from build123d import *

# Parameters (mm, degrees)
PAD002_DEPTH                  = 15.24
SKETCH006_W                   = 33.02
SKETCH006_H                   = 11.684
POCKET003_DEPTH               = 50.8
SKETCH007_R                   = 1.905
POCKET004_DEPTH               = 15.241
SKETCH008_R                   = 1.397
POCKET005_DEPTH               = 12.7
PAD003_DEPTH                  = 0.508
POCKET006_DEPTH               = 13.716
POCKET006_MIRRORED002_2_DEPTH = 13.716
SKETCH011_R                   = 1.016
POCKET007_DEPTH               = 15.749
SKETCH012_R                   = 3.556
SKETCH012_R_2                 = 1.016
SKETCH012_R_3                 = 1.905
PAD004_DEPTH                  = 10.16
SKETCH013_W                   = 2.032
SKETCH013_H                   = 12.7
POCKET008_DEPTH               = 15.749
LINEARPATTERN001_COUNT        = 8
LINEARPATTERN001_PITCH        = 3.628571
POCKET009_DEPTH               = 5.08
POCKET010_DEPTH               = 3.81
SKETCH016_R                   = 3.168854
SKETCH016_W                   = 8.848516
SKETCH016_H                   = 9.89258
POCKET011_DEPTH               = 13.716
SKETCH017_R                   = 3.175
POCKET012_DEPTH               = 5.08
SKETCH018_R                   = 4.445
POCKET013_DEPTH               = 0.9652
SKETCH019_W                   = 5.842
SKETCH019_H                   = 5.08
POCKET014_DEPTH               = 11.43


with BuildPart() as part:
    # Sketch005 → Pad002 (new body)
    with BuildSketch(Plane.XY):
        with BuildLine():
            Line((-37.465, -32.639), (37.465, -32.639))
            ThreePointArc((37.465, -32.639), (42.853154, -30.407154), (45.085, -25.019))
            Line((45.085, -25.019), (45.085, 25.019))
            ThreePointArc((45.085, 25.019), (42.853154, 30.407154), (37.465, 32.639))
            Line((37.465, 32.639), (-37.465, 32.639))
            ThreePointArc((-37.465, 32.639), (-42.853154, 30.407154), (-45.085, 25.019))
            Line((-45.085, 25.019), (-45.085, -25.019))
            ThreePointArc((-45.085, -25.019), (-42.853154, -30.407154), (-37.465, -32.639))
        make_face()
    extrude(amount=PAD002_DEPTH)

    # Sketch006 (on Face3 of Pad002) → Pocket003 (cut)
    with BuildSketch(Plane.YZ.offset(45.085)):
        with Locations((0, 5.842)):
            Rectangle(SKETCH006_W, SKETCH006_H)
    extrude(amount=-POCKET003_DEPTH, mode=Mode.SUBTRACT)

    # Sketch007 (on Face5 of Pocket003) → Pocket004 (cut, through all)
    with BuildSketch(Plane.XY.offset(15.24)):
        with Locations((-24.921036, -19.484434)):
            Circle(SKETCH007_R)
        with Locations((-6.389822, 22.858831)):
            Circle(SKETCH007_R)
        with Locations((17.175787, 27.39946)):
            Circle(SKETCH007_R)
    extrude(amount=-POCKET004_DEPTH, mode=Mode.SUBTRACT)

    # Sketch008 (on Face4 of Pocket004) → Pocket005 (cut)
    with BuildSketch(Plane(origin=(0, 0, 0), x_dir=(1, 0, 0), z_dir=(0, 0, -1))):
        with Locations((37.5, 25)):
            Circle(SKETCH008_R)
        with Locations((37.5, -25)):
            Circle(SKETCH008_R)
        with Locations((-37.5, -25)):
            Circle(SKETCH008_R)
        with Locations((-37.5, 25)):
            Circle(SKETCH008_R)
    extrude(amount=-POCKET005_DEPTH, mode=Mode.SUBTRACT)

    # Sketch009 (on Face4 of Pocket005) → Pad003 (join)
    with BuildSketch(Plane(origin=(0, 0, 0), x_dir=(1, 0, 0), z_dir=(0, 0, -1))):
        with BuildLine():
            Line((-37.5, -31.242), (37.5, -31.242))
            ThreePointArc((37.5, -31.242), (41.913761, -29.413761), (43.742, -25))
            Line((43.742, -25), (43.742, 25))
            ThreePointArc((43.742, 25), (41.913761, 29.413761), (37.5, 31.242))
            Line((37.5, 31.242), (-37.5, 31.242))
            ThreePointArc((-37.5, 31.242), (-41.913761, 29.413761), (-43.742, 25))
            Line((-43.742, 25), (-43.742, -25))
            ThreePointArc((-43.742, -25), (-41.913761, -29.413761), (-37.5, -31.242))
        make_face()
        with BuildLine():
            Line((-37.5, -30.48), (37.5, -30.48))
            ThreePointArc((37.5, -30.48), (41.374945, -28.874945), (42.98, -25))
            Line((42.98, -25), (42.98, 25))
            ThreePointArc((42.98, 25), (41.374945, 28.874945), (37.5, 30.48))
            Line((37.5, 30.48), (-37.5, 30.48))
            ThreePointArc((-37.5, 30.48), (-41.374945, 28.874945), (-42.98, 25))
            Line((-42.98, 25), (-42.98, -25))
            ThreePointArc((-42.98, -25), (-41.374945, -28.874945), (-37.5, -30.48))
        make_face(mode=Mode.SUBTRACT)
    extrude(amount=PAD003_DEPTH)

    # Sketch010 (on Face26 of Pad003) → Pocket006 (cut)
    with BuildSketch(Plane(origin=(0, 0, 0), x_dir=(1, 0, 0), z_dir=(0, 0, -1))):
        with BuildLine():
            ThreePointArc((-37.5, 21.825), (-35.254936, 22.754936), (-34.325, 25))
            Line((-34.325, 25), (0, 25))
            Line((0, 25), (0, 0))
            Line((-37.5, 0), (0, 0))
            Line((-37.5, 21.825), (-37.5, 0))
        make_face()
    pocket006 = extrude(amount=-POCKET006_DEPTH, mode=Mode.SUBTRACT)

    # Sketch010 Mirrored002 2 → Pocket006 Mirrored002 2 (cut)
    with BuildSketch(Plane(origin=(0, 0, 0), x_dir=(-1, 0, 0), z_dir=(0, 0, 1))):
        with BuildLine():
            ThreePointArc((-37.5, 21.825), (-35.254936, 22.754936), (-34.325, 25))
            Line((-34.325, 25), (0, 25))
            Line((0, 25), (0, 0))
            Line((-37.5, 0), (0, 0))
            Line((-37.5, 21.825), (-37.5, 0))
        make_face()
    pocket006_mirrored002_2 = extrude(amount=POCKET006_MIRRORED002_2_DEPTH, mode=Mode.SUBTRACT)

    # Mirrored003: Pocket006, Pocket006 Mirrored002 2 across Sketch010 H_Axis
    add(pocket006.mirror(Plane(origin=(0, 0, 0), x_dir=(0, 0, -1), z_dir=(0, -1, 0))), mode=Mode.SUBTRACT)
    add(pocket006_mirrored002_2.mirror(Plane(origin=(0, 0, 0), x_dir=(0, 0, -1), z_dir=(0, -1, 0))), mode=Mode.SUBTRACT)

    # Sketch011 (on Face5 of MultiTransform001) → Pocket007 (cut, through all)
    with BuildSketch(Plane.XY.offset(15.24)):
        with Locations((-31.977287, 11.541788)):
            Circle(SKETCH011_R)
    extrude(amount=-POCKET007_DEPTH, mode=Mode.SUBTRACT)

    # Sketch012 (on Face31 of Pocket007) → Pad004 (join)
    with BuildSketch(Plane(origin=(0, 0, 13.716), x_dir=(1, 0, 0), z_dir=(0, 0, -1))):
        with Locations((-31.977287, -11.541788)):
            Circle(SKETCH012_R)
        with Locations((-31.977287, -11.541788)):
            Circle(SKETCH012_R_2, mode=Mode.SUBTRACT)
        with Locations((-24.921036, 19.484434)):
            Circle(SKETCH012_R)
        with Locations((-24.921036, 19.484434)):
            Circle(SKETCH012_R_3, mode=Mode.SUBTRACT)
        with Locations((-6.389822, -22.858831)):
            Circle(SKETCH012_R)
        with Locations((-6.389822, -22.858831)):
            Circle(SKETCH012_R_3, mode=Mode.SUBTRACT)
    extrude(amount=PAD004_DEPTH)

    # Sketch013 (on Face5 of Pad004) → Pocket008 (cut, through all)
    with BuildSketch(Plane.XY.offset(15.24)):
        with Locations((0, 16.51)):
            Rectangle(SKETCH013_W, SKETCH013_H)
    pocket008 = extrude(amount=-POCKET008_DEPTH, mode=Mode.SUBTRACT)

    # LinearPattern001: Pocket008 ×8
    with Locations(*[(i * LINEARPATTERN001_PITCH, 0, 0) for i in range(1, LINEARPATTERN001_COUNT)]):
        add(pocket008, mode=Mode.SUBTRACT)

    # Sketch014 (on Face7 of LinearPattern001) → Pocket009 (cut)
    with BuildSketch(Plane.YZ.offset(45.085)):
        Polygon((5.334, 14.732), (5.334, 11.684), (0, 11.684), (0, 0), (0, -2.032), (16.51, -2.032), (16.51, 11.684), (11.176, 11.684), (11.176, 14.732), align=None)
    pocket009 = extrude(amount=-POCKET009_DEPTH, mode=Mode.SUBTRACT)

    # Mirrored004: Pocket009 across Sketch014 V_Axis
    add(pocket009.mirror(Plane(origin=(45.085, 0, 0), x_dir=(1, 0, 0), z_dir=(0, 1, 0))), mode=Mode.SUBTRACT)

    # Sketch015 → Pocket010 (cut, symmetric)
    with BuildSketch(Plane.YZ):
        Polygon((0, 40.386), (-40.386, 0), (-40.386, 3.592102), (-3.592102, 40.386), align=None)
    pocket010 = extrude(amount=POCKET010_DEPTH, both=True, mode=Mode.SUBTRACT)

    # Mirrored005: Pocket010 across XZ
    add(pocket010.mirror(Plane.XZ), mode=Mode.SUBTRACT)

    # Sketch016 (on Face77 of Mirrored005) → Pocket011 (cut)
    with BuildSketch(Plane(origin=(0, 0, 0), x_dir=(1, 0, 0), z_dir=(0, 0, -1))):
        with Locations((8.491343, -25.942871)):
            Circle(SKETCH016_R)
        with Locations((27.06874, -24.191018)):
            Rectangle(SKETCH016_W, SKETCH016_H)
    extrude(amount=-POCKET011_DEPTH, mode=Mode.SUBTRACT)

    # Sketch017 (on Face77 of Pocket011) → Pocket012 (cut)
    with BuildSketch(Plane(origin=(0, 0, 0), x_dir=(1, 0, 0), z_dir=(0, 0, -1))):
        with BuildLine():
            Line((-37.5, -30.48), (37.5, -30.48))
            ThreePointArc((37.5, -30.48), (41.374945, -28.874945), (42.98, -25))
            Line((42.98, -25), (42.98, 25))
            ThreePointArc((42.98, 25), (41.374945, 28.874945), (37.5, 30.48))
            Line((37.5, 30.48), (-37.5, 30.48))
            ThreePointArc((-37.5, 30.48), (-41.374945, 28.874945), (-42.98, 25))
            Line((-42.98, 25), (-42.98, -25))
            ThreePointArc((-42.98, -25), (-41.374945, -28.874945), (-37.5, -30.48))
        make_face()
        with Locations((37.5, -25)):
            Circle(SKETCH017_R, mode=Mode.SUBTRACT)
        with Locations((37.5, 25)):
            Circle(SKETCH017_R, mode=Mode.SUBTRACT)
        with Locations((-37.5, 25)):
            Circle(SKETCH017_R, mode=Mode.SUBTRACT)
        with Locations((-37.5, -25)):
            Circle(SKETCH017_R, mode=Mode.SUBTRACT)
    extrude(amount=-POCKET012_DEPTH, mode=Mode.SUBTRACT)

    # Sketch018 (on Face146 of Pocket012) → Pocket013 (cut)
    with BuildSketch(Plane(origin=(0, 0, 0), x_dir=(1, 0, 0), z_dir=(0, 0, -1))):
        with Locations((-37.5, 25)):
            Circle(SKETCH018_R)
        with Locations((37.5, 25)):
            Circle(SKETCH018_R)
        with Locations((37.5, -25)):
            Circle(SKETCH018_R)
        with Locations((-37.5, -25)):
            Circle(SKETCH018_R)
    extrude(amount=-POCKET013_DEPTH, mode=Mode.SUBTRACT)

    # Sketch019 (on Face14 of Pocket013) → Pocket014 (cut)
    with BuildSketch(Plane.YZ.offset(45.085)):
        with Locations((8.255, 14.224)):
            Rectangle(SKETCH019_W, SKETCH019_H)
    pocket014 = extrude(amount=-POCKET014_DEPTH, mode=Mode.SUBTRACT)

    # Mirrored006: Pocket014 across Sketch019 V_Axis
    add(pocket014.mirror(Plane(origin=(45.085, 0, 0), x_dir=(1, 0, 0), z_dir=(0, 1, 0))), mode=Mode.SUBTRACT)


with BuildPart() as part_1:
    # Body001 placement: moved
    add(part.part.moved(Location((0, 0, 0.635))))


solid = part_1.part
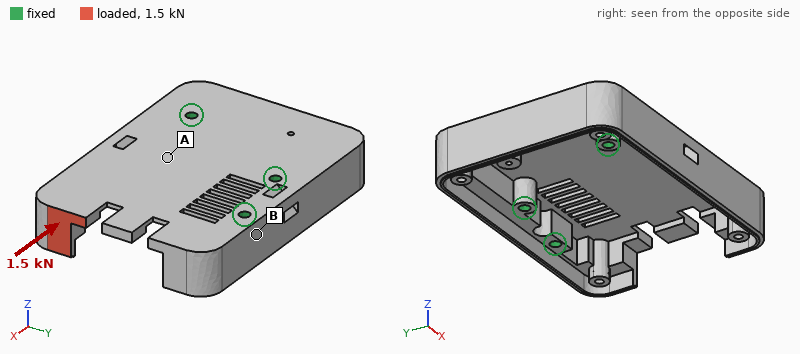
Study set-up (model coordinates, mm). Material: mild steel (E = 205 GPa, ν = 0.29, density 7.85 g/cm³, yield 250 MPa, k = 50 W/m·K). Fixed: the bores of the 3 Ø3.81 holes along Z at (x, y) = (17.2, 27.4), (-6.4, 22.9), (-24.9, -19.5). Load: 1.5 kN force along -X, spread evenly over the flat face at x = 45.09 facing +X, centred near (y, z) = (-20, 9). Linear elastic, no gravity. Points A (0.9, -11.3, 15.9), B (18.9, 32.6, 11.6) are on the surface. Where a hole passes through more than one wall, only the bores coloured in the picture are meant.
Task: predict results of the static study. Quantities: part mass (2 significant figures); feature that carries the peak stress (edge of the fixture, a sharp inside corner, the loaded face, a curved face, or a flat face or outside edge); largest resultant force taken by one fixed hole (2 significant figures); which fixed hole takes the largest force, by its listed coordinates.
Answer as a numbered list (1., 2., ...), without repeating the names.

1. 220 g
2. a flat face or outside edge
3. 1.4 kN
4. (-24.9, -19.5)
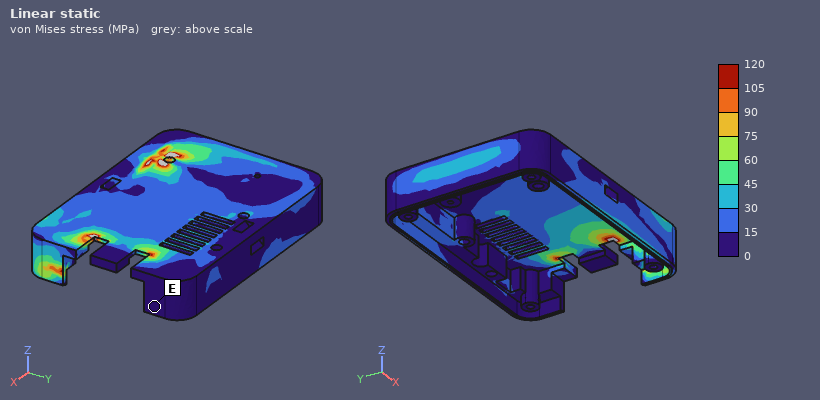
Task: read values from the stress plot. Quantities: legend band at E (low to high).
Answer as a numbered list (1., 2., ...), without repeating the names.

1. 0 to 15 MPa
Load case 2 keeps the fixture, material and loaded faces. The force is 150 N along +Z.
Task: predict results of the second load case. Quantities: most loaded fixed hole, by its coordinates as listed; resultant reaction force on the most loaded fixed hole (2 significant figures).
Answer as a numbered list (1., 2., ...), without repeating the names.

1. (-6.4, 22.9)
2. 320 N
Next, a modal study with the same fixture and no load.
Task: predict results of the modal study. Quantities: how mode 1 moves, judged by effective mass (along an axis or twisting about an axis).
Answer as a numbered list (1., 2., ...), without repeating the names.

1. along Z
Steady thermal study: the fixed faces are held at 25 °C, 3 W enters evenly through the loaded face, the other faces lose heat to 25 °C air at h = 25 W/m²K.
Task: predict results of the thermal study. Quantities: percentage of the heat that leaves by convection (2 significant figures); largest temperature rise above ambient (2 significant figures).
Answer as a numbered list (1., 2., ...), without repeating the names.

1. 62 %
2. 24 K
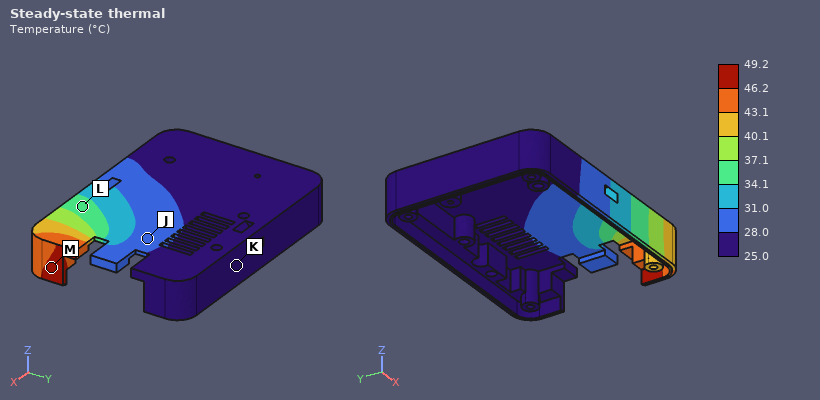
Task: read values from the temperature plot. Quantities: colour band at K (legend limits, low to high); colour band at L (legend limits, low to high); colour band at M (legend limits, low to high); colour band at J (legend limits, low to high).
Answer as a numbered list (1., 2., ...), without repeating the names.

1. 25.0 to 28.0 °C
2. 34.1 to 37.1 °C
3. 46.2 to 49.2 °C
4. 28.0 to 31.0 °C
